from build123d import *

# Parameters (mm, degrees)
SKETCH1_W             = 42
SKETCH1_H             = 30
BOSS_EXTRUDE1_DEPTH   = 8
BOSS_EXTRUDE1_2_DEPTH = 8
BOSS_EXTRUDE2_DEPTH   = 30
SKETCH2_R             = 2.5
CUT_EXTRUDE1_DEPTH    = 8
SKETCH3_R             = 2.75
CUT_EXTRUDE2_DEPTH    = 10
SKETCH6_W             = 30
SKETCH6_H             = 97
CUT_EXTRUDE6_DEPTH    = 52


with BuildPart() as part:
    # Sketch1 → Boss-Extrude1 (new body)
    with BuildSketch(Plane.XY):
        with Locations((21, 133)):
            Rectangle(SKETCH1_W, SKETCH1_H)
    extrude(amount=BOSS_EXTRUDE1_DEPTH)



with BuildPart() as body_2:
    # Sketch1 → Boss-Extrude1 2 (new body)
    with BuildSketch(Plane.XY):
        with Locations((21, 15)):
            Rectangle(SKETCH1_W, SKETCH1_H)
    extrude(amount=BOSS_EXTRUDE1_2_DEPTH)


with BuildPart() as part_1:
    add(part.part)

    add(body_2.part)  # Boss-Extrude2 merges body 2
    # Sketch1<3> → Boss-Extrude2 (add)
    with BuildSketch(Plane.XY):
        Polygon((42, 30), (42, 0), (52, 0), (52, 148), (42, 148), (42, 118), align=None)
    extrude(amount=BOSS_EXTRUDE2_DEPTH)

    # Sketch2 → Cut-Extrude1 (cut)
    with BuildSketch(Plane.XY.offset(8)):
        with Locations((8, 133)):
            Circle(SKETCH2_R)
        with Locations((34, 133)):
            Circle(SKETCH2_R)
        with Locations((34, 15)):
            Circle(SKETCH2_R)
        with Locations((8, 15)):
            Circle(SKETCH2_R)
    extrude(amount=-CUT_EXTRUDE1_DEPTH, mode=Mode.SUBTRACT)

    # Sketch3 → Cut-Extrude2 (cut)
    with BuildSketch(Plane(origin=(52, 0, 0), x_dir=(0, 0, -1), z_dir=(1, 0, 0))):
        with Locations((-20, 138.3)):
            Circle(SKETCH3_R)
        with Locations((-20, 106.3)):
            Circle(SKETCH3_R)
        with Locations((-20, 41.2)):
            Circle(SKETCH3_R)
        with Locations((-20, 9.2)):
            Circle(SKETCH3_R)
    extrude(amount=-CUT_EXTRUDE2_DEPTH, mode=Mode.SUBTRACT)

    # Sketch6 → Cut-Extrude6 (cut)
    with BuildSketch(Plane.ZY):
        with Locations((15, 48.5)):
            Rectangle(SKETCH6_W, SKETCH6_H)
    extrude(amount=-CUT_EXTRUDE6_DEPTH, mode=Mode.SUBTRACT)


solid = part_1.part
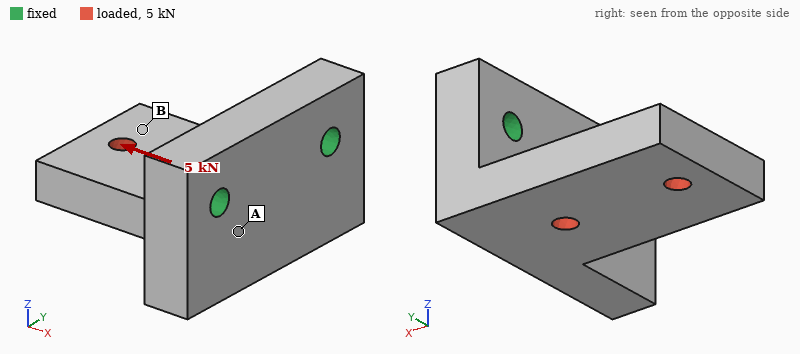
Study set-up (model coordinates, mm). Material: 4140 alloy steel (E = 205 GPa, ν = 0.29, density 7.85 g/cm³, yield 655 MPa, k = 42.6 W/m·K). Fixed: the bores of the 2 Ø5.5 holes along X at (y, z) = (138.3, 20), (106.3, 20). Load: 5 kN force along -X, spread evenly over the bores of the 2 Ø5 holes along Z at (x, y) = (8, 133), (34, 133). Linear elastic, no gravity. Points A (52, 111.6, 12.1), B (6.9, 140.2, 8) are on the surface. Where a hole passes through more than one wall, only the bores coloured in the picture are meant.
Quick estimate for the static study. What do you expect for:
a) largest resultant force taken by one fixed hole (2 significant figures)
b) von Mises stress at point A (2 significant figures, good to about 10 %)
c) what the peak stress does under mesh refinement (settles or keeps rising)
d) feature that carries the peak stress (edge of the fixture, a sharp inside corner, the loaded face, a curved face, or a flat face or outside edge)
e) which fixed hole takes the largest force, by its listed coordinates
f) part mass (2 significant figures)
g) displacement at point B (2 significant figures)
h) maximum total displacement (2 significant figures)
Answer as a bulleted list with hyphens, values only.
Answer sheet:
- 3.9 kN
- 48 MPa
- keeps rising
- edge of the fixture
- (138.3, 20)
- 190 g
- 49 µm
- 60 µm
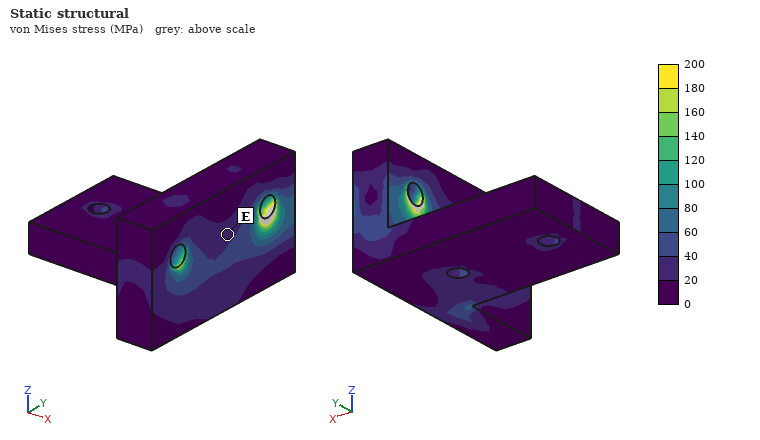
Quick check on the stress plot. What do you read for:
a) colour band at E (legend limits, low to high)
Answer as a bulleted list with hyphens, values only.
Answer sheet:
- 20 to 40 MPa
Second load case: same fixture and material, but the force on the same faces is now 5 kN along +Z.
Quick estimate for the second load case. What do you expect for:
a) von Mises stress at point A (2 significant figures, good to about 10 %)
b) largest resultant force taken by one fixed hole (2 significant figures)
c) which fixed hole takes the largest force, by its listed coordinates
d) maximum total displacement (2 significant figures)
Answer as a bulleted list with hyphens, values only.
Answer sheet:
- 110 MPa
- 4.2 kN
- (138.3, 20)
- 0.40 mm
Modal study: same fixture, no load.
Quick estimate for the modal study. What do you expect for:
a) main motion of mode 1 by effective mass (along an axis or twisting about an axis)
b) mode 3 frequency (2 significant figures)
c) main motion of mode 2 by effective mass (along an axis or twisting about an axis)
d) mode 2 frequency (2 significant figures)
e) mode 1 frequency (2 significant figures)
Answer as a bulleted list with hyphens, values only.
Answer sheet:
- along Z
- 8900 Hz
- along Y
- 5200 Hz
- 2500 Hz
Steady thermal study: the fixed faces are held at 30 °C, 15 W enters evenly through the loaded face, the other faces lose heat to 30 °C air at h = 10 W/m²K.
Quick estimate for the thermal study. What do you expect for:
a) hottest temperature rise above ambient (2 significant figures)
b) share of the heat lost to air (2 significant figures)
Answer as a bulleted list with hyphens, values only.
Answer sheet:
- 50 K
- 9.5 %
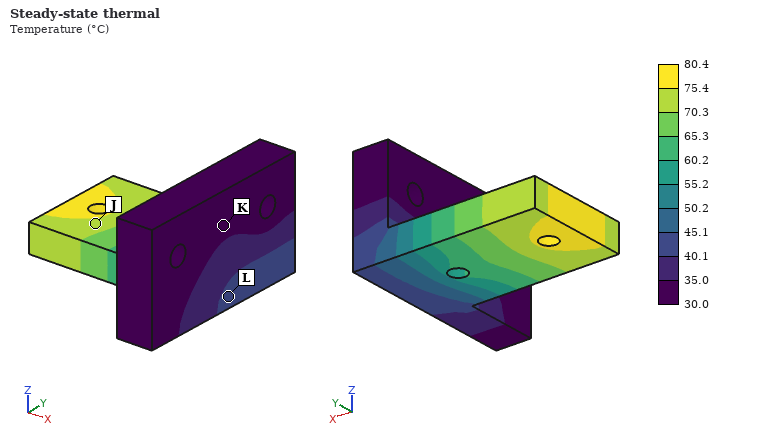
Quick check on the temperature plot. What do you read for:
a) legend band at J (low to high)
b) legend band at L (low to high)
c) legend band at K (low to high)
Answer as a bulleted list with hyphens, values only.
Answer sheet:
- 70.3 to 75.4 °C
- 40.1 to 45.1 °C
- 30.0 to 35.0 °C
